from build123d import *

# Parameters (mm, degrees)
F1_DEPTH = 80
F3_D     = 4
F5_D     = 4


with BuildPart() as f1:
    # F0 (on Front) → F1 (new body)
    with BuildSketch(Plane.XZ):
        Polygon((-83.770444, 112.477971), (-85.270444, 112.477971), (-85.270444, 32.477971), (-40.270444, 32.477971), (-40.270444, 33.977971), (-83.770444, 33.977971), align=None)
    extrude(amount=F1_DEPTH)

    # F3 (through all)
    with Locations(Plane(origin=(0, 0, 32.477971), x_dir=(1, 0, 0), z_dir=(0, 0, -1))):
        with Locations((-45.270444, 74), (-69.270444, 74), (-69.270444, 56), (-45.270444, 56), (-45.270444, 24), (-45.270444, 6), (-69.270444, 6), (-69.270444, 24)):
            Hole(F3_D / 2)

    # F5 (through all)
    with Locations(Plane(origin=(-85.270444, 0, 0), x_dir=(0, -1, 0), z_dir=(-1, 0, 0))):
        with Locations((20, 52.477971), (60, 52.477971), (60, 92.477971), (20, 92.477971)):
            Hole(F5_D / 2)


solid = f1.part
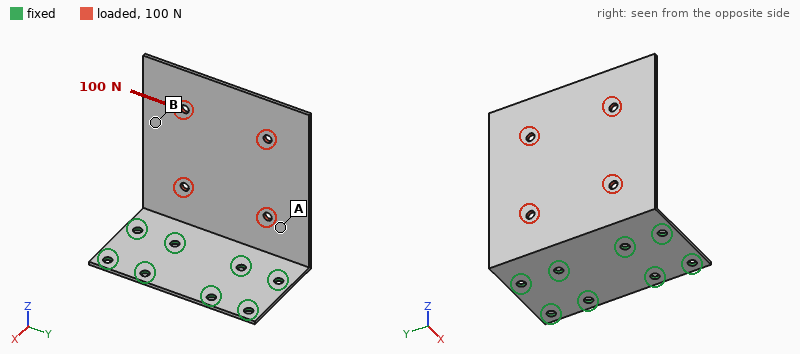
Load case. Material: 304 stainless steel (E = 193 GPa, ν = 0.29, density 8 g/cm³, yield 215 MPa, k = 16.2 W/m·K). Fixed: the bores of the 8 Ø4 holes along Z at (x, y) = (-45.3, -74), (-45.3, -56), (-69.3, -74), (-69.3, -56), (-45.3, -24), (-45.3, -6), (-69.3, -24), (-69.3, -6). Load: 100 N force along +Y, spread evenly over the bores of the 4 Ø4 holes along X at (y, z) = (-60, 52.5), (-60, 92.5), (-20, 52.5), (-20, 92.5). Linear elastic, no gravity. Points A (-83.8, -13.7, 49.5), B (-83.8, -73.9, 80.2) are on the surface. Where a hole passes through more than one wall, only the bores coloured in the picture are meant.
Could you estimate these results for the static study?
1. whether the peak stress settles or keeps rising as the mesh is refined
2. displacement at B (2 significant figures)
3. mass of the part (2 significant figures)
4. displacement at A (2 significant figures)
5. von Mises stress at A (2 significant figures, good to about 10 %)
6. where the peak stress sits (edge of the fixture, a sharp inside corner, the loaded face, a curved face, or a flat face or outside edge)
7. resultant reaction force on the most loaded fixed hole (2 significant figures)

keeps rising
0.075 mm
120 g
0.038 mm
11 MPa
edge of the fixture
55 N
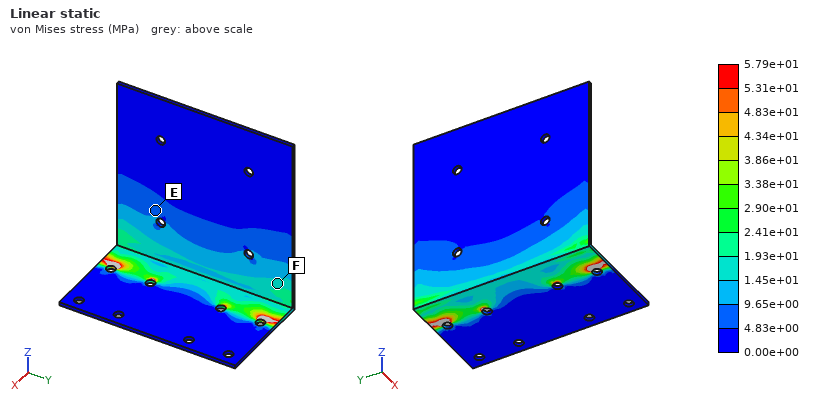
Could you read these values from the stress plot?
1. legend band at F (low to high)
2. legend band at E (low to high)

1.45e+01 to 1.93e+01 MPa
4.83e+00 to 9.65e+00 MPa
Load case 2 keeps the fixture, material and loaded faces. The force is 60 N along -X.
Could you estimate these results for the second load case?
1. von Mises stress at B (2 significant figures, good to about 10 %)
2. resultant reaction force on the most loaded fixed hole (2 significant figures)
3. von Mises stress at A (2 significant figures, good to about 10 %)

13 MPa
23 N
43 MPa
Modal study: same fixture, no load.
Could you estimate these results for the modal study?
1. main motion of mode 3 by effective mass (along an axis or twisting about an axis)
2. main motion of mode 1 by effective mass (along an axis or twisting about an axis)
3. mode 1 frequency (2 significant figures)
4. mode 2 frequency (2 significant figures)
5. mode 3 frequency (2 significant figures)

along Y
along X
150 Hz
420 Hz
780 Hz
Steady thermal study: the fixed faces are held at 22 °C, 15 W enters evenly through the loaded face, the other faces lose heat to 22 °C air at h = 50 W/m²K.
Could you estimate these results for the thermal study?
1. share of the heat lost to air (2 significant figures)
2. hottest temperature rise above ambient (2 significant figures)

95 %
63 K
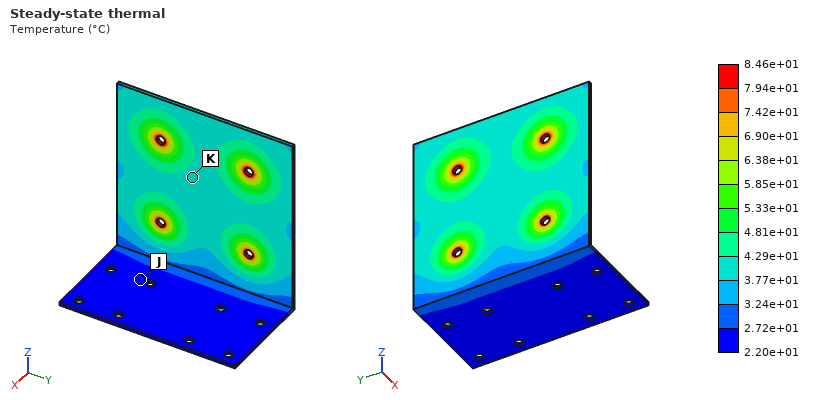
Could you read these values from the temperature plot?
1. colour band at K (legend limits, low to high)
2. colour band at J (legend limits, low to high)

3.77e+01 to 4.29e+01 °C
2.20e+01 to 2.72e+01 °C
